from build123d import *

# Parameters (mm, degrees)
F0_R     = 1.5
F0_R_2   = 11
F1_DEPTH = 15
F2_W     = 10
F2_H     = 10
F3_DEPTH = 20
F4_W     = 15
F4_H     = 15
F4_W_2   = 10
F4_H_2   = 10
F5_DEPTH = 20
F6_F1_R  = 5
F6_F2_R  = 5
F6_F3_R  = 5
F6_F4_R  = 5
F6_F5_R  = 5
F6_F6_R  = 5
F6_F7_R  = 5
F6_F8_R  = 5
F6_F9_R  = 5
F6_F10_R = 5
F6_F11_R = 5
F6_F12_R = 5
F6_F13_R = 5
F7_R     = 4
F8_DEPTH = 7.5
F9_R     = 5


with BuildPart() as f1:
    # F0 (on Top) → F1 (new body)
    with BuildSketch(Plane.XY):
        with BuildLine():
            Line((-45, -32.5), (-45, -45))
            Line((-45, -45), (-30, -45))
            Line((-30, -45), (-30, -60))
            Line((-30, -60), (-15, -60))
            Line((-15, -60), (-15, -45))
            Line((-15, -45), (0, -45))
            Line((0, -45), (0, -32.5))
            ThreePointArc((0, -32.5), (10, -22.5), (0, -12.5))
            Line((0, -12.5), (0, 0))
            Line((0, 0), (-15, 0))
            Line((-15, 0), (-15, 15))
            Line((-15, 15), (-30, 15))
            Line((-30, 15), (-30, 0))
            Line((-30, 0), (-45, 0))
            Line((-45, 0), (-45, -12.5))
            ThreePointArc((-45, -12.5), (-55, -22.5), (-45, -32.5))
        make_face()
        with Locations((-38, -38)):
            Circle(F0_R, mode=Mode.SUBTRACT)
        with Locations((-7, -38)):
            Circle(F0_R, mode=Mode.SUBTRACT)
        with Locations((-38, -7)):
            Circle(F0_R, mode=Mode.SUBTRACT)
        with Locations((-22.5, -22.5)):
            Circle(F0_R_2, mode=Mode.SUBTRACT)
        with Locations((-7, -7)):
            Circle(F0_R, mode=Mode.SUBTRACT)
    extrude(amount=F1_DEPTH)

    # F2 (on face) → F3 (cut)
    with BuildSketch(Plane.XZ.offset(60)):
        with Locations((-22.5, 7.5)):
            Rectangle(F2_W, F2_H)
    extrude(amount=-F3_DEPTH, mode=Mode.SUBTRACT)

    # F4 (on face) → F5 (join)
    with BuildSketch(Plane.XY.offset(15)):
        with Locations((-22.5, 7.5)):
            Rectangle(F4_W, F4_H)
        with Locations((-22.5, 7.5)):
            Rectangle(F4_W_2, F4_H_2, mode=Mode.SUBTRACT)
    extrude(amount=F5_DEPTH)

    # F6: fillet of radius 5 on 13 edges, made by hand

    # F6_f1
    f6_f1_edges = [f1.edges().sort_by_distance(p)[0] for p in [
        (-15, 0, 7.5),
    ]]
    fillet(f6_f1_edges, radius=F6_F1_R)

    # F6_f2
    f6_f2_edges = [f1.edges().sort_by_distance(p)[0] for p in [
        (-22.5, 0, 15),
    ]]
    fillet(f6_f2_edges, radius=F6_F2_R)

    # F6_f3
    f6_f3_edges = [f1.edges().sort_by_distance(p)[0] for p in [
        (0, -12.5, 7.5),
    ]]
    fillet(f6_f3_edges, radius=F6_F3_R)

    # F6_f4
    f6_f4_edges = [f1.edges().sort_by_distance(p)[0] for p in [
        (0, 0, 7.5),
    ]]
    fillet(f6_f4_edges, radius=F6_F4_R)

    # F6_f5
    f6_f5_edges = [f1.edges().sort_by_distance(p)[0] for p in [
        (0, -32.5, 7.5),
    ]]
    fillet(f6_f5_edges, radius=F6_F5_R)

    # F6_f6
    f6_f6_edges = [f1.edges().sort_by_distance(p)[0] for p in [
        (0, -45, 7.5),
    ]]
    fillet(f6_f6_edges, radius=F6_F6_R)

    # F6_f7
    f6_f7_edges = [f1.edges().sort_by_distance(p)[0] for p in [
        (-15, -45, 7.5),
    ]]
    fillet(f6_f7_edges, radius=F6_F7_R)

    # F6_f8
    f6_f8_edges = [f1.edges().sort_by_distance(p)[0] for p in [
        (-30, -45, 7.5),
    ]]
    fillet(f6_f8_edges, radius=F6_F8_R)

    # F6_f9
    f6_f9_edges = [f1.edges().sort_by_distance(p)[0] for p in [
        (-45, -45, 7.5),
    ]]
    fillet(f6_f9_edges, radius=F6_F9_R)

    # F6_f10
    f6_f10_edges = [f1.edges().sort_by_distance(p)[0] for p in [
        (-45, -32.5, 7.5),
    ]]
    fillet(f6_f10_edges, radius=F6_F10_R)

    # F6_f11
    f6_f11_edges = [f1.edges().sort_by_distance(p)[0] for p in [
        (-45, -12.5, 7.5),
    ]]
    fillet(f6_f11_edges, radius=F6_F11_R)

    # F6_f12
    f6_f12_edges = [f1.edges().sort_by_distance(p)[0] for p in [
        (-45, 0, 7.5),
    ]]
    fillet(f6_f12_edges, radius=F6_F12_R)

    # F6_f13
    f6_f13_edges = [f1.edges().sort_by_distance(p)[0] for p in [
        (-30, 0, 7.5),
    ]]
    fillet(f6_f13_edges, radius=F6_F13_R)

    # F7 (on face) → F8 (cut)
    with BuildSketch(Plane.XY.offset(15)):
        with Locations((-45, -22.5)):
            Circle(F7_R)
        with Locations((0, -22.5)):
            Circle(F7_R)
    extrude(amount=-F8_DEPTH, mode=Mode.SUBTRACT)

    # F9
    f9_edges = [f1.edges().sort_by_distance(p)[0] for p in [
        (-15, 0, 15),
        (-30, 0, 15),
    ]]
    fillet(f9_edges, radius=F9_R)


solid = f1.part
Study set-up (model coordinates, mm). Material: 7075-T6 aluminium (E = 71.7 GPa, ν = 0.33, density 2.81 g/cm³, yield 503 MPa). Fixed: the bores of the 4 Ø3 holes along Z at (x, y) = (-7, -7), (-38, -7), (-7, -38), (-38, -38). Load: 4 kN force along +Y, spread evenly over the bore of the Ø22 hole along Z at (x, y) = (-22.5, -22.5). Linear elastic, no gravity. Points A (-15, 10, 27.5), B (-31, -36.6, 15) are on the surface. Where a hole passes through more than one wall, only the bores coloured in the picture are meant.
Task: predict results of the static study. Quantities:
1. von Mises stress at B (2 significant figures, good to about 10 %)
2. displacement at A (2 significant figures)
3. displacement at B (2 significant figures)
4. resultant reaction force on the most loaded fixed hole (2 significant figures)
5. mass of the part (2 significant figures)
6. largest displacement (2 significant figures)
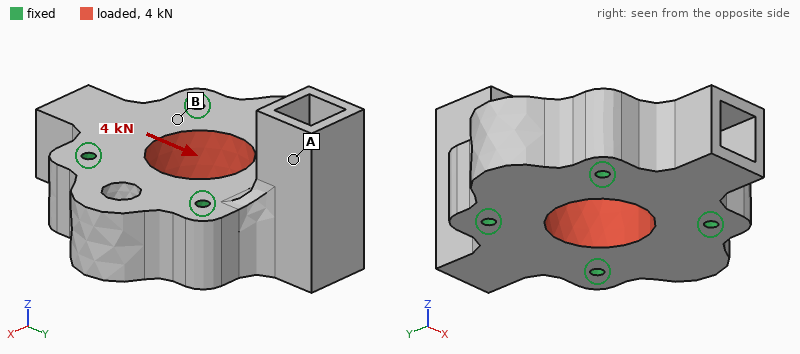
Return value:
4.3 MPa
1.1 µm
1.1 µm
1.0 kN
100 g
2.1 µm
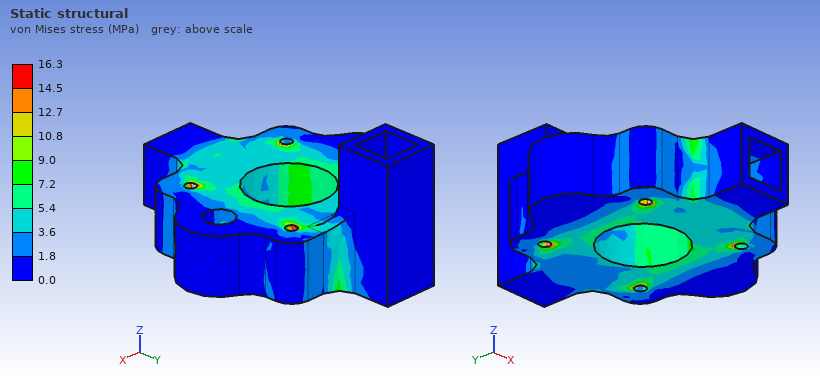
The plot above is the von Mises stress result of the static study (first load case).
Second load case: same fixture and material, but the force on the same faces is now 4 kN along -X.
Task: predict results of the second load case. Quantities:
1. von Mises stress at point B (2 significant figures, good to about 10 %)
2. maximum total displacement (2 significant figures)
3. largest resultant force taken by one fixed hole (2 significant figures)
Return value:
4.7 MPa
2.0 µm
1.0 kN
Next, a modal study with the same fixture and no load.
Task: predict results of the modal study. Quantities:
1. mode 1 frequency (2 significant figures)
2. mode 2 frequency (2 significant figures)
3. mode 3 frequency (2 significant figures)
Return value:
9400 Hz
14 kHz
19 kHz
